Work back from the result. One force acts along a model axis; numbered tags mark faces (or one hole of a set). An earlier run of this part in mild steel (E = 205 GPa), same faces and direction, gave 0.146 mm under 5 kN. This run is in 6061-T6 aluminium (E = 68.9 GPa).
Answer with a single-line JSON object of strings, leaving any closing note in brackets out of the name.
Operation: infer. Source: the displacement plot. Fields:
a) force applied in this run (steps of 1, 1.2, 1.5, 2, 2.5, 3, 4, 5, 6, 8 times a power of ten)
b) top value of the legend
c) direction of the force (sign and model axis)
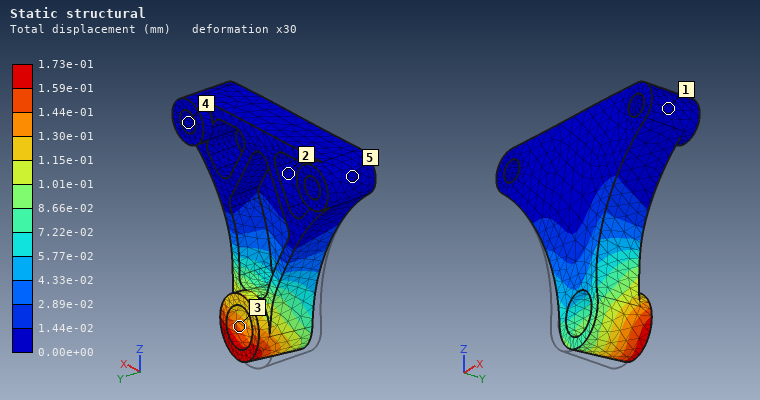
{"force applied in this run": "2 kN", "top value of the legend": "1.73e-01 mm", "direction of the force": "+X"}
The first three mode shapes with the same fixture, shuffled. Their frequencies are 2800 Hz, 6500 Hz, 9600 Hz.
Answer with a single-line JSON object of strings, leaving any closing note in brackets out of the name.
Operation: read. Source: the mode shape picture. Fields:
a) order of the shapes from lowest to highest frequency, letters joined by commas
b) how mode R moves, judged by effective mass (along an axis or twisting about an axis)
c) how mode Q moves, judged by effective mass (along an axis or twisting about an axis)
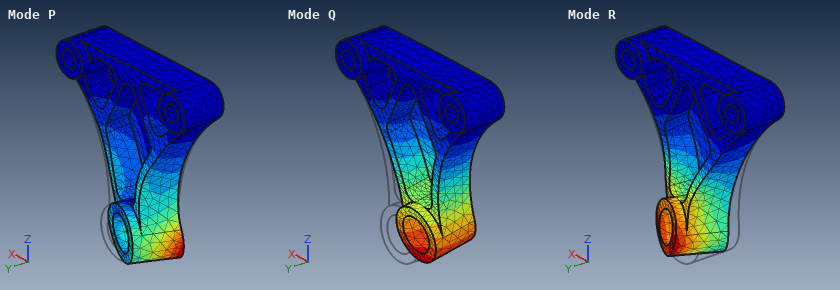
{"order of the shapes from lowest to highest frequency, letters joined by commas": "Q, R, P", "how mode R moves, judged by effective mass": "along X", "how mode Q moves, judged by effective mass": "along Y"}
